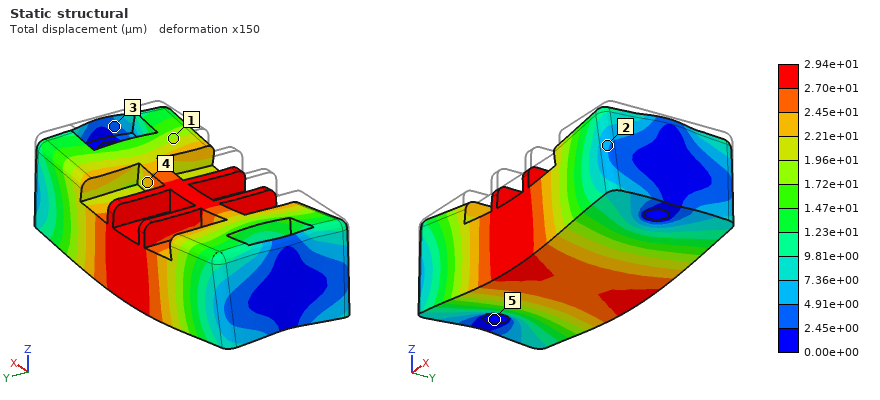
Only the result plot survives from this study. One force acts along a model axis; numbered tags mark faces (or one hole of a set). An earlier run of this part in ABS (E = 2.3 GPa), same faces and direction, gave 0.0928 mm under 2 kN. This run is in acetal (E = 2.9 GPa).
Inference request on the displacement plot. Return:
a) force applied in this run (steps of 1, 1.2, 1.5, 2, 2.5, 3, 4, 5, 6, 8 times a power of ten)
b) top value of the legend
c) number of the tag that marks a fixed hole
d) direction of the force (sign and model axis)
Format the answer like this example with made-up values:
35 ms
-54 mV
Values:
800 N
2.94e+01 µm
5
-Z
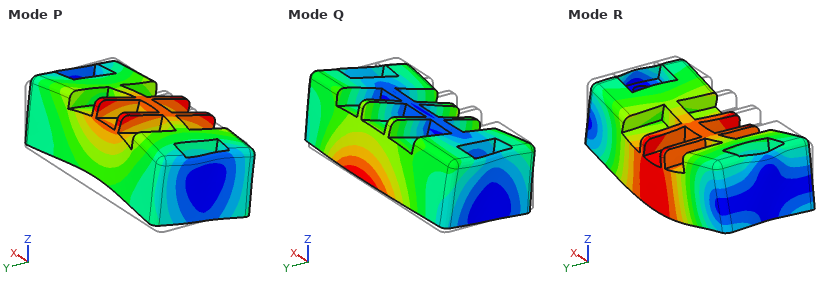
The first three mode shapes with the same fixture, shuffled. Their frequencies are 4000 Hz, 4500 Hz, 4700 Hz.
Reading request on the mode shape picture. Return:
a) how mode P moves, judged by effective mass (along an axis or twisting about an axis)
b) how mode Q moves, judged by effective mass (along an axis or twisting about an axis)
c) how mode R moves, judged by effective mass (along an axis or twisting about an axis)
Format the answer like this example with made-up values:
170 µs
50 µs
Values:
along Y
along Y
along Z
